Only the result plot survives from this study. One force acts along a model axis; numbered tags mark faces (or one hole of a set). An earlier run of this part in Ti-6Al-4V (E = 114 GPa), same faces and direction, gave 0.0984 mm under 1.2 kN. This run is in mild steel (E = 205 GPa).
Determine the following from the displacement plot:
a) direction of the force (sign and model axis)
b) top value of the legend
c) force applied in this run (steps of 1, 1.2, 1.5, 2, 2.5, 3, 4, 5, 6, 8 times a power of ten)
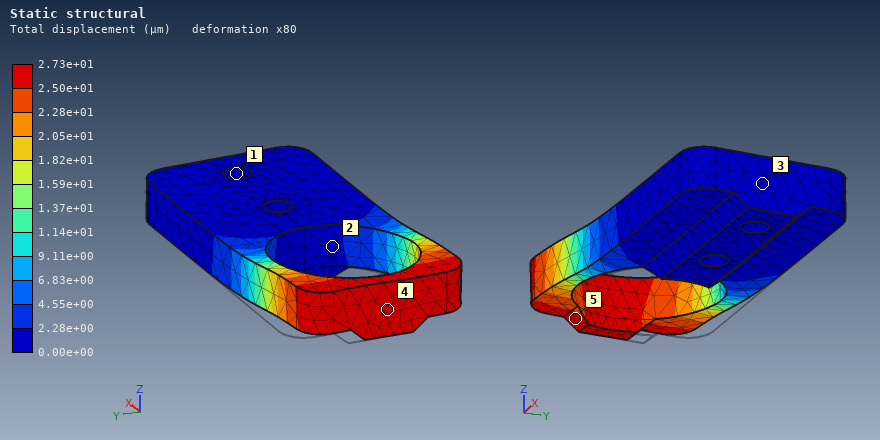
-Y
2.73e+01 µm
600 N
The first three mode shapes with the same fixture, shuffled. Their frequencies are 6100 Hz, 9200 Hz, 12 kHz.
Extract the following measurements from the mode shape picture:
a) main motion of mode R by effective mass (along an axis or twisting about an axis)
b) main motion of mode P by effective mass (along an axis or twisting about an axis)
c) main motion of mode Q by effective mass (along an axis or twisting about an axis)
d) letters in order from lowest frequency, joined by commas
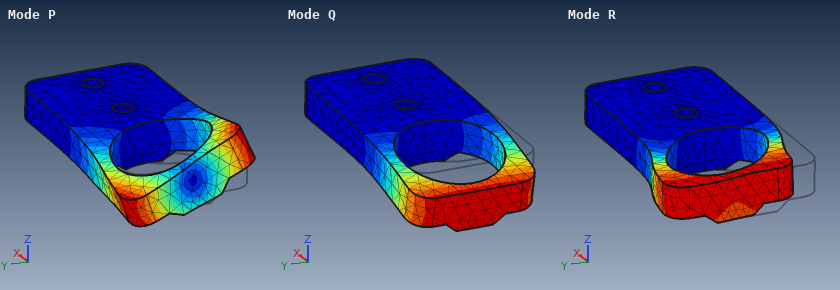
along Y
twisting about X
along Z
Q, R, P
